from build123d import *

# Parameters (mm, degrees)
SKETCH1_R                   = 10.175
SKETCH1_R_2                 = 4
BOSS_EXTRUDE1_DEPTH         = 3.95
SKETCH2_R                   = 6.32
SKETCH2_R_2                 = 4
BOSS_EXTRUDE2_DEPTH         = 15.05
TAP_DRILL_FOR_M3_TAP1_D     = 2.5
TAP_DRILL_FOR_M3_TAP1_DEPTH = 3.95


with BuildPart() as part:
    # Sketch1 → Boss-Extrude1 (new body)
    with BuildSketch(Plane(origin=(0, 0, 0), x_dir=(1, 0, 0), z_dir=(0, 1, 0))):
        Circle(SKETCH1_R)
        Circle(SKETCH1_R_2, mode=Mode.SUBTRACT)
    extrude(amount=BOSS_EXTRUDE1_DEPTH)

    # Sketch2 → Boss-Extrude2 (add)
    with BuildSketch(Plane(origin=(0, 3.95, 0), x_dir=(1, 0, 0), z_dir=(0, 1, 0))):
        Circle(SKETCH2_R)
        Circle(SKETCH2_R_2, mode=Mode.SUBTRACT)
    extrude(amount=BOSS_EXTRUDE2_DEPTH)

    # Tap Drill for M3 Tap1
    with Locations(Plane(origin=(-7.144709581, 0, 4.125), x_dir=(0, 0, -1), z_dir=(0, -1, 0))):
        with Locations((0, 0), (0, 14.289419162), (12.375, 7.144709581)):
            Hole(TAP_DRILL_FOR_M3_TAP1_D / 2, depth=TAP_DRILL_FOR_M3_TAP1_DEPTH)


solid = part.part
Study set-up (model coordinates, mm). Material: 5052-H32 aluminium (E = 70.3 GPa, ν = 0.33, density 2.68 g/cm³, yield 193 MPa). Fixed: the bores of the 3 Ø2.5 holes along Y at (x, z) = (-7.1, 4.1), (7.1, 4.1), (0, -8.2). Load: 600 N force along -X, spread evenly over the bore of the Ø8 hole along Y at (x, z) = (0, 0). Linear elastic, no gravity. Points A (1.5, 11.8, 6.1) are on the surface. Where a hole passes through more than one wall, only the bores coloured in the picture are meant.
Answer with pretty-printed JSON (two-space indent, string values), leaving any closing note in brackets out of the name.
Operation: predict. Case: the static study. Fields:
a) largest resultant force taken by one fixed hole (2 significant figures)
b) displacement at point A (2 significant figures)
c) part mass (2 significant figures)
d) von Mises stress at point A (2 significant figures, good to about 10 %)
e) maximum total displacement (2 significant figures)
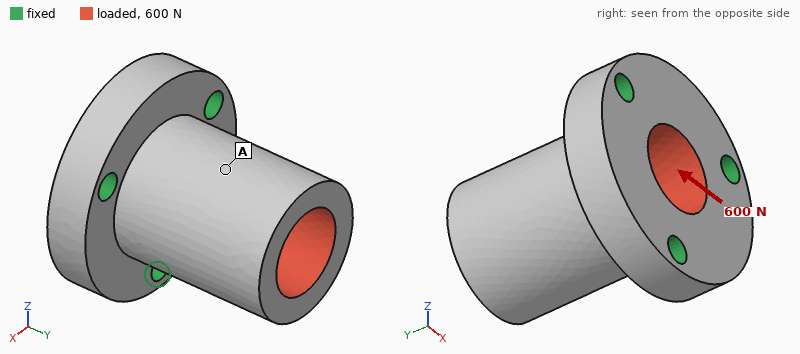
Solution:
{
  "largest resultant force taken by one fixed hole": "360 N",
  "displacement at point A": "6.3 µm",
  "part mass": "5.8 g",
  "von Mises stress at point A": "8.7 MPa",
  "maximum total displacement": "12 µm"
}
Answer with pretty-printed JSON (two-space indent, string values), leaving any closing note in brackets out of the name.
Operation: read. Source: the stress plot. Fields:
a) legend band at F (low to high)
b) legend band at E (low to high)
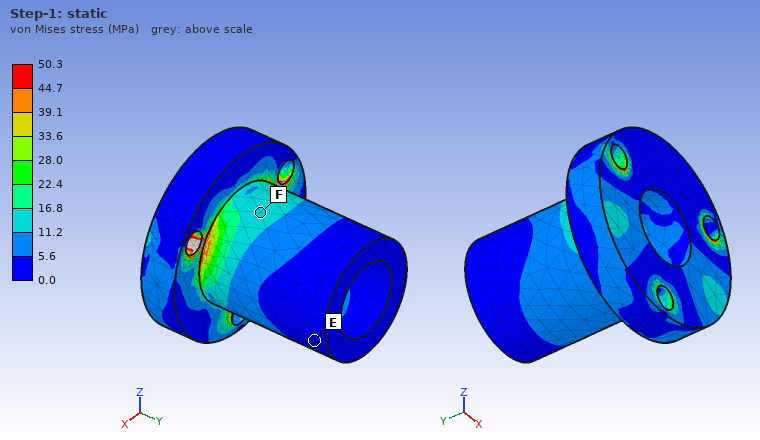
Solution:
{
  "legend band at F": "11.2 to 16.8 MPa",
  "legend band at E": "0.0 to 5.6 MPa"
}
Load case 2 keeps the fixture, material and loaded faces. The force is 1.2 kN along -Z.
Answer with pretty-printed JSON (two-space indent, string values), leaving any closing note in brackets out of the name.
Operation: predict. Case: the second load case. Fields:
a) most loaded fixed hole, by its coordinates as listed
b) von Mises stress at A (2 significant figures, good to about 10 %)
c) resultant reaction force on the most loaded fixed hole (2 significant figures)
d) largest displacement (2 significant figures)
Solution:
{
  "most loaded fixed hole, by its coordinates as listed": "(0, -8.2)",
  "von Mises stress at A": "12 MPa",
  "resultant reaction force on the most loaded fixed hole": "810 N",
  "largest displacement": "24 µm"
}
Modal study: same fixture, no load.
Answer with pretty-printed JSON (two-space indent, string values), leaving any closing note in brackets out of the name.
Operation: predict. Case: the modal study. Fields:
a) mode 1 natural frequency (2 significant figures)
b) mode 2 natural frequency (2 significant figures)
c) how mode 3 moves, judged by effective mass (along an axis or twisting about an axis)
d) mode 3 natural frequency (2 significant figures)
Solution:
{
  "mode 1 natural frequency": "21 kHz",
  "mode 2 natural frequency": "22 kHz",
  "how mode 3 moves, judged by effective mass": "twisting about Y",
  "mode 3 natural frequency": "47 kHz"
}
